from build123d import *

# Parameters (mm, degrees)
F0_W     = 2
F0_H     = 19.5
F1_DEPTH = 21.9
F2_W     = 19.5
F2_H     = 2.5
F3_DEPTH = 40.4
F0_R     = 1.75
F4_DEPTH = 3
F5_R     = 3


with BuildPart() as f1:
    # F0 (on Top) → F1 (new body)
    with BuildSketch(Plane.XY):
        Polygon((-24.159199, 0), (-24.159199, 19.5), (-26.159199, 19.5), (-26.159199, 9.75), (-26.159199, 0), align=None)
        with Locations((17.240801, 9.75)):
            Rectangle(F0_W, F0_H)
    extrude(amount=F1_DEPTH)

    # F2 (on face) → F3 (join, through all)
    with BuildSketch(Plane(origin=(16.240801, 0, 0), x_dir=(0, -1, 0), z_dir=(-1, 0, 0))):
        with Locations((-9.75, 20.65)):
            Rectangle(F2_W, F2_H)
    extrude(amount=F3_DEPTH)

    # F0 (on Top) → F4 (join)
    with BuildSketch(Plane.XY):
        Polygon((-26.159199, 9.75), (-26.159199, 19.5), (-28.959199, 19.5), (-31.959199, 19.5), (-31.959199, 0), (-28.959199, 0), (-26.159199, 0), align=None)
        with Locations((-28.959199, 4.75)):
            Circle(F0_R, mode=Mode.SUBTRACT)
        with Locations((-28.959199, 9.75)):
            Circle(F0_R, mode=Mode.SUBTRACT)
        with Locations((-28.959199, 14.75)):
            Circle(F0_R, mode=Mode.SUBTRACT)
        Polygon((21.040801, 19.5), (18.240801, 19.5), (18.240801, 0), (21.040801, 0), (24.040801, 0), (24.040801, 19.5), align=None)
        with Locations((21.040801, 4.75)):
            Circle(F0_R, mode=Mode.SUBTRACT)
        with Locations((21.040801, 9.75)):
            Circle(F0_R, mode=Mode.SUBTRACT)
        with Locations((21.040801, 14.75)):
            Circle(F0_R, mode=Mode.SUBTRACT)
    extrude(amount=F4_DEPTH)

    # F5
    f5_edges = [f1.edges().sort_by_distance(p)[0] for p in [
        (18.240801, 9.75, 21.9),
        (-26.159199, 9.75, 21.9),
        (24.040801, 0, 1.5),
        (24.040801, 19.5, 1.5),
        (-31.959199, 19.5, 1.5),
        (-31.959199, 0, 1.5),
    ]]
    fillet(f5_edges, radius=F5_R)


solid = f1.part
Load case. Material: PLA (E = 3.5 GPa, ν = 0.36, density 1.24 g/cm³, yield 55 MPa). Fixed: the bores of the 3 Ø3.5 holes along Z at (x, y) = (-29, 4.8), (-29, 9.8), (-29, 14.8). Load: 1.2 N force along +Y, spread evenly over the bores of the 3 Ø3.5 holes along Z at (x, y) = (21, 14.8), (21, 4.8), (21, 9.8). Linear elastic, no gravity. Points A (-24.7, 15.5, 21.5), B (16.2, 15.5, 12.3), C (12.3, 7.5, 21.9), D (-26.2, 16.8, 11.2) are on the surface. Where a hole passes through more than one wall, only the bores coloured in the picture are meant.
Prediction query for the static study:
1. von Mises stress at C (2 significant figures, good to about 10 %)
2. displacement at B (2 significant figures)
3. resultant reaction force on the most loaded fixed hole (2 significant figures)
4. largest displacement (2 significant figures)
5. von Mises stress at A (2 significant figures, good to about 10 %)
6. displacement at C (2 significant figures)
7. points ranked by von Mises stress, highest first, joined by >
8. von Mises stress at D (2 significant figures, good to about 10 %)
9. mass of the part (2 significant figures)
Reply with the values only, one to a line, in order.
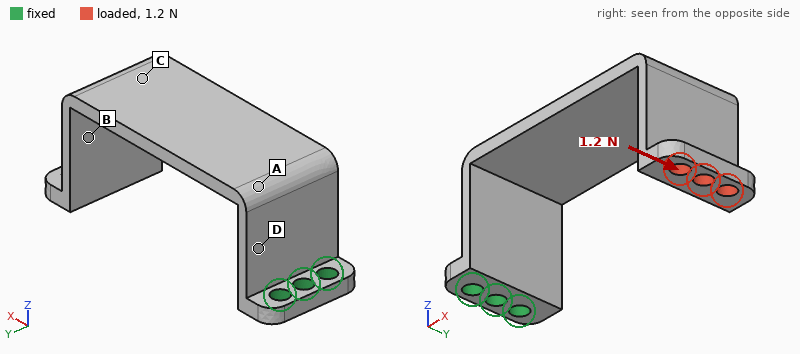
0.84 MPa
0.54 mm
4.5 N
0.74 mm
2.0 MPa
0.40 mm
D > A > C > B
3.0 MPa
5.1 g
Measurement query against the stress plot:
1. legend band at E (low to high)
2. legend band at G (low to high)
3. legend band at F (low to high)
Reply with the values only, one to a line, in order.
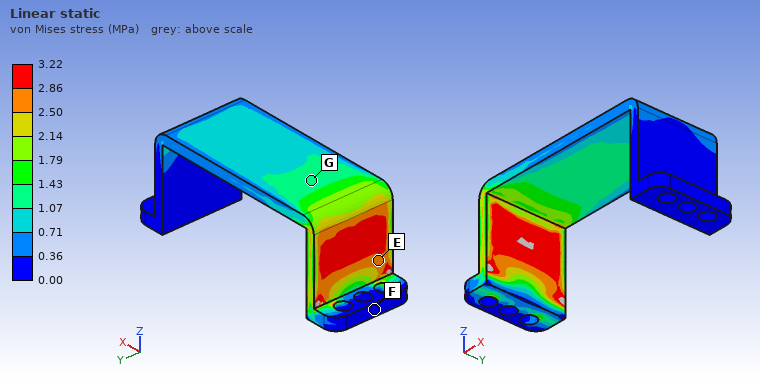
2.50 to 2.86 MPa
1.07 to 1.43 MPa
0.00 to 0.36 MPa
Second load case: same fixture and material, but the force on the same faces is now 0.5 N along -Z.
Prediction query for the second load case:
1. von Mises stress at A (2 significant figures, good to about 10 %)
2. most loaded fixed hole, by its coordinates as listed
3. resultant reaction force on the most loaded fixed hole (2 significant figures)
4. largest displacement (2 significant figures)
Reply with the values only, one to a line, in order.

0.84 MPa
(-29, 9.8)
0.61 N
0.68 mm
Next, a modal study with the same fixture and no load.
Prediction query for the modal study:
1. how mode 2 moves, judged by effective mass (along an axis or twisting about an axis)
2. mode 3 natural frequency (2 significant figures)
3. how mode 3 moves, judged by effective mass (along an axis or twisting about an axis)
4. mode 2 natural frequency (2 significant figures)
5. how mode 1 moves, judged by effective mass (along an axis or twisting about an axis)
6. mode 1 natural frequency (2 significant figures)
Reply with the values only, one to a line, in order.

along Y
410 Hz
along X
170 Hz
along Z
110 Hz
